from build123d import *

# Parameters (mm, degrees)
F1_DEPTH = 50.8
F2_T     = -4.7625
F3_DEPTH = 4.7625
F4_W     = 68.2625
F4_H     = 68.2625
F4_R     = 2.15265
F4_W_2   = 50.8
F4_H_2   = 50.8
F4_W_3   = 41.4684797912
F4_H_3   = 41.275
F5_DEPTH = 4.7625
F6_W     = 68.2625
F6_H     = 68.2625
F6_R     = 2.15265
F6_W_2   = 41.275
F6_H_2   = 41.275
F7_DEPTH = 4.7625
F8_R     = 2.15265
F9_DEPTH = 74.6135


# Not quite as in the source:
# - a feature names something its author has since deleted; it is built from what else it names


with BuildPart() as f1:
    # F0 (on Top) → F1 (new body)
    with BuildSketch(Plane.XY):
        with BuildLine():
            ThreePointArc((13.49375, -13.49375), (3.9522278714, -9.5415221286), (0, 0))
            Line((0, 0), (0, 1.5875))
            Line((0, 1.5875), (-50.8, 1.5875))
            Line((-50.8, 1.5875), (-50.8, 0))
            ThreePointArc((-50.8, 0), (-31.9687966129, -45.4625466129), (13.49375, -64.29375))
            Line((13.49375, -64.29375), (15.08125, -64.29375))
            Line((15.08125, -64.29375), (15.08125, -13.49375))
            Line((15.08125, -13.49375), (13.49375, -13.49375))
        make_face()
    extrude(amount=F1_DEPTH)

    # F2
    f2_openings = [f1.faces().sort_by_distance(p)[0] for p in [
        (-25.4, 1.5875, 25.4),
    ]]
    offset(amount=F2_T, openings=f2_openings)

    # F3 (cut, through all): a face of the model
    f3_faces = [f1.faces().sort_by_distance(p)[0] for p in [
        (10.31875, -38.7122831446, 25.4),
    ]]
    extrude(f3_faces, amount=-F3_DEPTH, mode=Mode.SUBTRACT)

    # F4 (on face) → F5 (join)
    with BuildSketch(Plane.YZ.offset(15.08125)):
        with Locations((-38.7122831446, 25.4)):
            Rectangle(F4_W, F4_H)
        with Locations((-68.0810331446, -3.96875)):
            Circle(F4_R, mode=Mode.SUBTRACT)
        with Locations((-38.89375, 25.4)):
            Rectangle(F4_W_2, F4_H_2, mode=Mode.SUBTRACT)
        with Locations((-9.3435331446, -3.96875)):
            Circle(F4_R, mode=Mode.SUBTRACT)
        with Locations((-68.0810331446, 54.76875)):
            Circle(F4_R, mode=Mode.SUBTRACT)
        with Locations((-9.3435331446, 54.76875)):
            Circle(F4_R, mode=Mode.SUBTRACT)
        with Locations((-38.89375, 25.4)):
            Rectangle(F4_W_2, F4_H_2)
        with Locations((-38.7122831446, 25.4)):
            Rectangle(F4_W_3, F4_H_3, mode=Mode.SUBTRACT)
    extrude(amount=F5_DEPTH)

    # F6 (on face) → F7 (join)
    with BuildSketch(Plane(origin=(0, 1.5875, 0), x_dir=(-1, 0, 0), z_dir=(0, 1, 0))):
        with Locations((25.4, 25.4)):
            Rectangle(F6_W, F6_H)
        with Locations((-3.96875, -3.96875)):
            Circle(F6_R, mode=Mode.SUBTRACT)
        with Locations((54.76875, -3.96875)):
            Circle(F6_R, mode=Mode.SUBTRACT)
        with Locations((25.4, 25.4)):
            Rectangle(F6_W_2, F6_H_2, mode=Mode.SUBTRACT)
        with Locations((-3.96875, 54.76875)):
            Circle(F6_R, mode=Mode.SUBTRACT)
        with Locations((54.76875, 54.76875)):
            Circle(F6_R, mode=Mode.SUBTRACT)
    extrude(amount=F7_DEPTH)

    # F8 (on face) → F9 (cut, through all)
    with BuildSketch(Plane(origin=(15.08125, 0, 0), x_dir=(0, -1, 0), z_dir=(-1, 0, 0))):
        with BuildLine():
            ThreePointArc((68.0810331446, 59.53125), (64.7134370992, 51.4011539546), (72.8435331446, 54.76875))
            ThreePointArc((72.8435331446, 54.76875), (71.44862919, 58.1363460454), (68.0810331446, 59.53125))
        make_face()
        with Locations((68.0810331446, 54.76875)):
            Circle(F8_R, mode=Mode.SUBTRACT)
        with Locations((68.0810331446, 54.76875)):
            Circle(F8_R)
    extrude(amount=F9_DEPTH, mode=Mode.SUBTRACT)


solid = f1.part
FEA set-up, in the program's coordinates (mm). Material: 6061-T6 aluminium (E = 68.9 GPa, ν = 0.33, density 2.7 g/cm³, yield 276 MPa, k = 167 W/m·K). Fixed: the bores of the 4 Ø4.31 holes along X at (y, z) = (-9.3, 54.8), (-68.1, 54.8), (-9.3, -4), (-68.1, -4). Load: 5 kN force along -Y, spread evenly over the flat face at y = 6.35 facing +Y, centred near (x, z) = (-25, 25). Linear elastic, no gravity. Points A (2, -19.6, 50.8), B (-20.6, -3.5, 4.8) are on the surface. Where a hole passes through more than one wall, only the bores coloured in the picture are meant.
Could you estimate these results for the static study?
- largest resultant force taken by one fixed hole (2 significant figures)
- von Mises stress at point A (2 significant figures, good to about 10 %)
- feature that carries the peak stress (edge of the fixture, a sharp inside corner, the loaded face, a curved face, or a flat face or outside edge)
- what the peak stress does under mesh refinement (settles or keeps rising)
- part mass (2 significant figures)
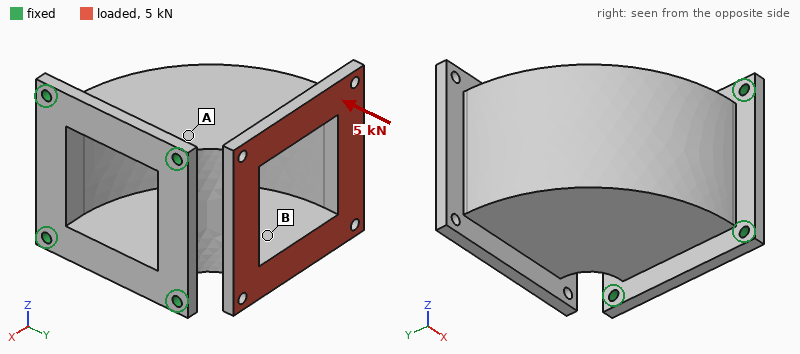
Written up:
2.5 kN
31 MPa
edge of the fixture
keeps rising
230 g
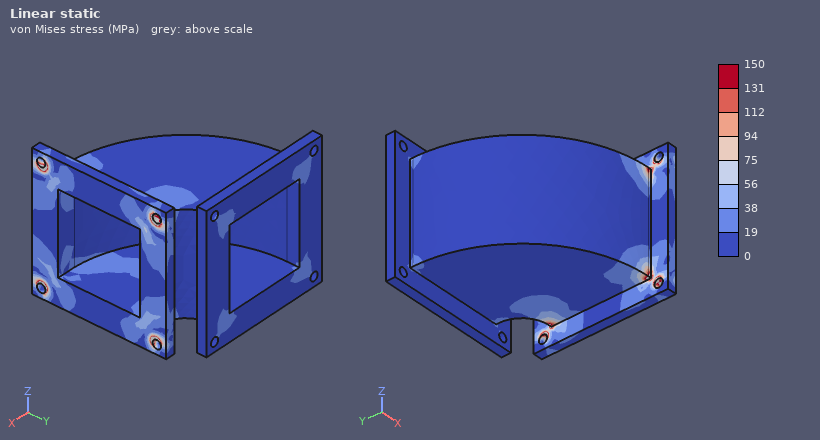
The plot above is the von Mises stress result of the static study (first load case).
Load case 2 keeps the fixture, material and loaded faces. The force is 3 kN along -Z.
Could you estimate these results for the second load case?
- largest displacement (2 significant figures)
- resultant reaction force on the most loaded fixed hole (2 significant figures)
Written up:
0.18 mm
2.2 kN
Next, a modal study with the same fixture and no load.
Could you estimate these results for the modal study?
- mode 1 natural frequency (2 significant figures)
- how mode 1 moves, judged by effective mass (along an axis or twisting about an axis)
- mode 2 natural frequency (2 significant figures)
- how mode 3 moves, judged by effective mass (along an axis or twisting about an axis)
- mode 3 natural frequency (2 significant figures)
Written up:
2400 Hz
along Z
2600 Hz
along X
5300 Hz
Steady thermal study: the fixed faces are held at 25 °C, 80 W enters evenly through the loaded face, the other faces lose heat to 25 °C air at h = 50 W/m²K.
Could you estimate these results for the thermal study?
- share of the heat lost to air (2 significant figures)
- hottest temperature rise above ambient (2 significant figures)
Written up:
42 %
39 K
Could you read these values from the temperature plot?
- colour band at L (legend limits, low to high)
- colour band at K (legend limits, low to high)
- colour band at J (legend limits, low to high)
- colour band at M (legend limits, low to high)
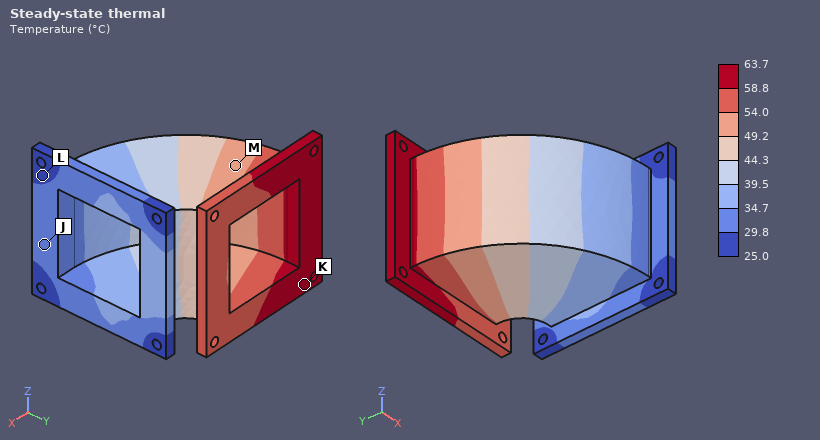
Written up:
25.0 to 29.8 °C
58.8 to 63.7 °C
29.8 to 34.7 °C
49.2 to 54.0 °C
